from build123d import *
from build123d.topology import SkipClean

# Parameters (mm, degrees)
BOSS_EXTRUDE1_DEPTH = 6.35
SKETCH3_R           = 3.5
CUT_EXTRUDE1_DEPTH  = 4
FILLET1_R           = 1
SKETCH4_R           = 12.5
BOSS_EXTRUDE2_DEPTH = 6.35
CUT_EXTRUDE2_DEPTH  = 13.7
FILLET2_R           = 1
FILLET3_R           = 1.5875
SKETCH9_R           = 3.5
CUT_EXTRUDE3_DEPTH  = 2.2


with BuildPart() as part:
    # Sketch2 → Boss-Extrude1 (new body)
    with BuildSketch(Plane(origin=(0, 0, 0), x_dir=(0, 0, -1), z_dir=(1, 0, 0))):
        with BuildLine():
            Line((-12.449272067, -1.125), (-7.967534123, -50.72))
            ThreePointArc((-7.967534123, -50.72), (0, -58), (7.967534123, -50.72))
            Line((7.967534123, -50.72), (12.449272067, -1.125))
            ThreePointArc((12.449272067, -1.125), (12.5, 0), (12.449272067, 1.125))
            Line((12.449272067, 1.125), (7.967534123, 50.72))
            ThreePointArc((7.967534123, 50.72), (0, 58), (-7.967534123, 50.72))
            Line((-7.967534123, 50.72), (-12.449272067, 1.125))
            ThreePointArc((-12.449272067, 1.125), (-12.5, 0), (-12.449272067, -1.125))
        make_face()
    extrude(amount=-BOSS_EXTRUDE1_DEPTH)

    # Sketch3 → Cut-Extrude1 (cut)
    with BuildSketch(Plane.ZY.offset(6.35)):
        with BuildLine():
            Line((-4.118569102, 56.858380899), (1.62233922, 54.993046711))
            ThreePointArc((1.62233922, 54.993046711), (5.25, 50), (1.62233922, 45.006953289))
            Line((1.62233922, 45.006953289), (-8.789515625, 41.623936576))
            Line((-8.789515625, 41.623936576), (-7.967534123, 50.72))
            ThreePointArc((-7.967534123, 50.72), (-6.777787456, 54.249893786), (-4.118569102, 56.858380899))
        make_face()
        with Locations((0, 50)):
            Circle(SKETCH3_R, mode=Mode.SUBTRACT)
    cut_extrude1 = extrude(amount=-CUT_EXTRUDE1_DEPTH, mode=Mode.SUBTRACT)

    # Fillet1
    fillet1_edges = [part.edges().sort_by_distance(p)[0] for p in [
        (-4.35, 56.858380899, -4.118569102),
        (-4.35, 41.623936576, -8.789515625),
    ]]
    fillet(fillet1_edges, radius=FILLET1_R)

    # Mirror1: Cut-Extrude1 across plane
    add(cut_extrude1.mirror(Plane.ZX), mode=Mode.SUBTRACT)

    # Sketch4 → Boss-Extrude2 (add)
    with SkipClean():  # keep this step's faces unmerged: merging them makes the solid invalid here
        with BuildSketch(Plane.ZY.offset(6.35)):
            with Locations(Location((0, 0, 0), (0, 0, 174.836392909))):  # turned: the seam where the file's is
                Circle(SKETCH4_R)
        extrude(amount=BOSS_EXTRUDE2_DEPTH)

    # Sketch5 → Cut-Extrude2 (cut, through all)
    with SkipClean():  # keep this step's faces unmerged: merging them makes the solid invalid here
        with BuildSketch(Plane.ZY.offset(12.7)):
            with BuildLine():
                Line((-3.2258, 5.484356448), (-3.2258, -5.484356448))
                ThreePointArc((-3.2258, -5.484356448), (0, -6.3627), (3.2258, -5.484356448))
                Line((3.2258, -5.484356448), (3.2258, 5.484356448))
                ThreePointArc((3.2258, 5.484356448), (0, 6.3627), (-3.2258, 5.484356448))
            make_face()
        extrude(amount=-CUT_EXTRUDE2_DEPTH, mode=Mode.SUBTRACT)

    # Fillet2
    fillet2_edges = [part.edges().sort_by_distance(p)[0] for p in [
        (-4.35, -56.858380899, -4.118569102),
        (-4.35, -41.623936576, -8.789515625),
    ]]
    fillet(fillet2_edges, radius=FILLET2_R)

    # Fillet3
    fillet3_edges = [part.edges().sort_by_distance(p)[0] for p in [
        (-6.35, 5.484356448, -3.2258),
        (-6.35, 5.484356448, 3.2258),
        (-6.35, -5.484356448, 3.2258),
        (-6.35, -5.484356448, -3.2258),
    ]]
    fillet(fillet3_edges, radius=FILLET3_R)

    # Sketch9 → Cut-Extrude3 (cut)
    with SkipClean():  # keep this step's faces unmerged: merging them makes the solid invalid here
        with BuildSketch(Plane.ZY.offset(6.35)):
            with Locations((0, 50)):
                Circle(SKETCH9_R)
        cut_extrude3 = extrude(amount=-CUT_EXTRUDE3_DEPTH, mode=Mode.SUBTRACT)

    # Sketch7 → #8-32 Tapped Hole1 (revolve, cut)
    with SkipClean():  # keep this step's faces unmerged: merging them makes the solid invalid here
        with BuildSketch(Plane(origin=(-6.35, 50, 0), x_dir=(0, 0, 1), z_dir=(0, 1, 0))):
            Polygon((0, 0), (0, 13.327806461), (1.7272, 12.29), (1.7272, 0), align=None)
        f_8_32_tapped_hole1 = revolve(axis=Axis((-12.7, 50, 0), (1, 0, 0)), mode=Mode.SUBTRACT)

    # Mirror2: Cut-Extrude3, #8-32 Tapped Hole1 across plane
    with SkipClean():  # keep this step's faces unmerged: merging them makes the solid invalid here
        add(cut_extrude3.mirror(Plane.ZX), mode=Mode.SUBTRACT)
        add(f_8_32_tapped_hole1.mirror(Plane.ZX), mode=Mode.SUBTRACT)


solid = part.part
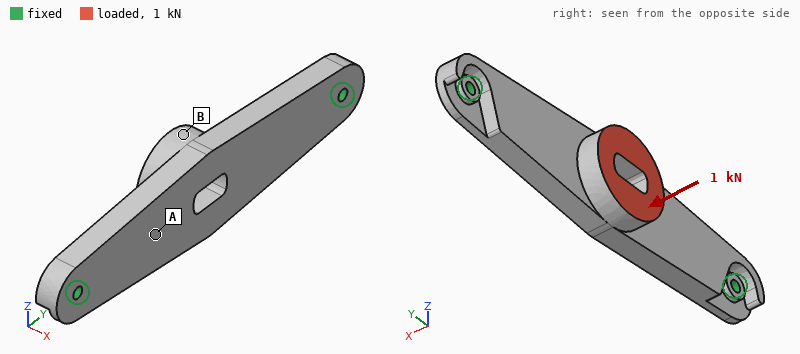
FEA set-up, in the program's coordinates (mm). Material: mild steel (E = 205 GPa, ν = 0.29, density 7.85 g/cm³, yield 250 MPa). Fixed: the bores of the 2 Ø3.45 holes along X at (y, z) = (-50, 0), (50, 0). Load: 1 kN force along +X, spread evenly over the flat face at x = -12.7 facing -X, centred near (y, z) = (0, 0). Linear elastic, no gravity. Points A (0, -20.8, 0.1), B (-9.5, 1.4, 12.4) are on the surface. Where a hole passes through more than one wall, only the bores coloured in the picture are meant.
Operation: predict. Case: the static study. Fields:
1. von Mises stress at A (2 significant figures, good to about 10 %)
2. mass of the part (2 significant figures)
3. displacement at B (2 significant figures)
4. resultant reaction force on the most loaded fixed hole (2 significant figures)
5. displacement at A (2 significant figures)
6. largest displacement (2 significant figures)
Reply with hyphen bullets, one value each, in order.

- 36 MPa
- 120 g
- 67 µm
- 1.5 kN
- 53 µm
- 67 µm
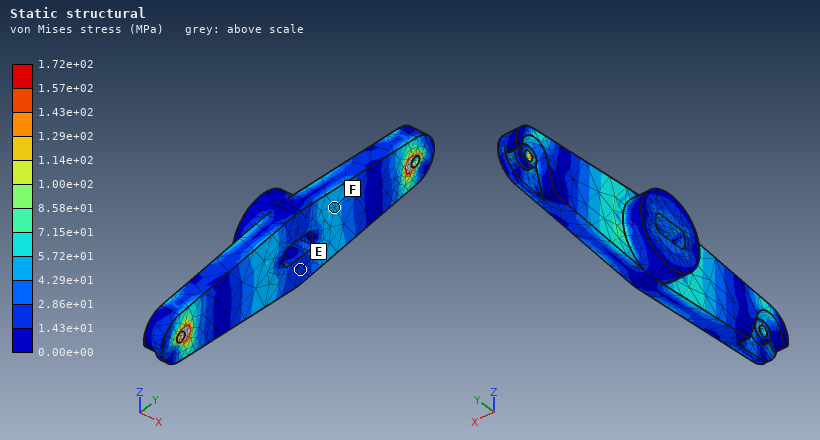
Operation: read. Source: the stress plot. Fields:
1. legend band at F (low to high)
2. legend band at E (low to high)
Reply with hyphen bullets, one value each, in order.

- 4.29e+01 to 5.72e+01 MPa
- 1.43e+01 to 2.86e+01 MPa
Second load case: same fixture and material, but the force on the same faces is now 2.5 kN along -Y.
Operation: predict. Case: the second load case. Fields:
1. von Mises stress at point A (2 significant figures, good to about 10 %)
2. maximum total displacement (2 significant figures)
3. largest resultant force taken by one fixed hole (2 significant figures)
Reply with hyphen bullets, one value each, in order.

- 24 MPa
- 16 µm
- 1.3 kN
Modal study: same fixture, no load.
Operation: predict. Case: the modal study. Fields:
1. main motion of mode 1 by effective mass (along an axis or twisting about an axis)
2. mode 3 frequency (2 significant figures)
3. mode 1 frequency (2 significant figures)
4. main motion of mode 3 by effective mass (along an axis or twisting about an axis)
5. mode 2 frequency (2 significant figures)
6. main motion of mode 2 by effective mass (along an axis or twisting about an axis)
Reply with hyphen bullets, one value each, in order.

- along X
- 5500 Hz
- 2300 Hz
- along Z
- 3300 Hz
- along Z
